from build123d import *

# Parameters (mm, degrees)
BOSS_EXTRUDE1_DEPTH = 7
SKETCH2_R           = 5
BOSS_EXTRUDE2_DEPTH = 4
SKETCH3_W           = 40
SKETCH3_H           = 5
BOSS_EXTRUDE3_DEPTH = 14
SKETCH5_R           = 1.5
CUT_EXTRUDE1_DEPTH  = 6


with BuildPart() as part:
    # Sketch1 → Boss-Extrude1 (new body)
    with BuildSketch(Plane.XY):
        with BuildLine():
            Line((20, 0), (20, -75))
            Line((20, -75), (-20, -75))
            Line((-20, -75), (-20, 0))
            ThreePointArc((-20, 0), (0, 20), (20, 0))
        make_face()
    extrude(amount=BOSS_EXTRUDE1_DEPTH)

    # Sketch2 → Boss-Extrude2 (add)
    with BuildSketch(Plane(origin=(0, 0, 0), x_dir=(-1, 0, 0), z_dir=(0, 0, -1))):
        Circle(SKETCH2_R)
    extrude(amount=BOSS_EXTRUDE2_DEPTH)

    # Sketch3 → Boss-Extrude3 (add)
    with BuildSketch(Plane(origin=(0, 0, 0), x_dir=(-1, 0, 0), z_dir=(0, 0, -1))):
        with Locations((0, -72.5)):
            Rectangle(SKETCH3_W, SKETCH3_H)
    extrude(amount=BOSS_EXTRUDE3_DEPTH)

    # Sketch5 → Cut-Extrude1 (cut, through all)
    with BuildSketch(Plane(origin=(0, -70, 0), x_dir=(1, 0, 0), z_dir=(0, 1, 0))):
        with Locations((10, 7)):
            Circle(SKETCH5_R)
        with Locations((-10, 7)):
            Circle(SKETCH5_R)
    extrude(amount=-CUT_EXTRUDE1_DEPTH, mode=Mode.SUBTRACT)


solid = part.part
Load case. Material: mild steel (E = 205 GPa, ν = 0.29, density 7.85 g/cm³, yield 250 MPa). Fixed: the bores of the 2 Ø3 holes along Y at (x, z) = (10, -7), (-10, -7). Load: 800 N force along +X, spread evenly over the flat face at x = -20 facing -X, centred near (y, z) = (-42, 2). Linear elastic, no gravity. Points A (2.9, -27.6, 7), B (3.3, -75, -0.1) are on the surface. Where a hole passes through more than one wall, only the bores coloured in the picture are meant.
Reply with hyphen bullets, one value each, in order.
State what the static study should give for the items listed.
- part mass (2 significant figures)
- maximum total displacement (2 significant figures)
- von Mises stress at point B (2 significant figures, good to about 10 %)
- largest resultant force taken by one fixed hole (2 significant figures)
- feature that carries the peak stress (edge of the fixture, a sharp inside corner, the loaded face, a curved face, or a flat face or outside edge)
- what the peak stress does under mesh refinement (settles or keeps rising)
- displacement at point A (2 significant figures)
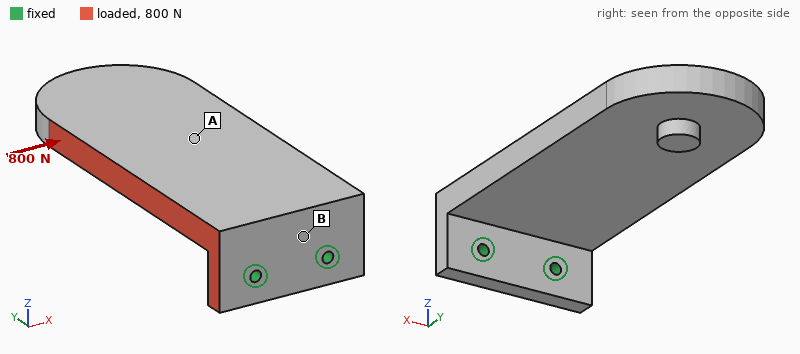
- 220 g
- 55 µm
- 28 MPa
- 1.2 kN
- edge of the fixture
- keeps rising
- 25 µm
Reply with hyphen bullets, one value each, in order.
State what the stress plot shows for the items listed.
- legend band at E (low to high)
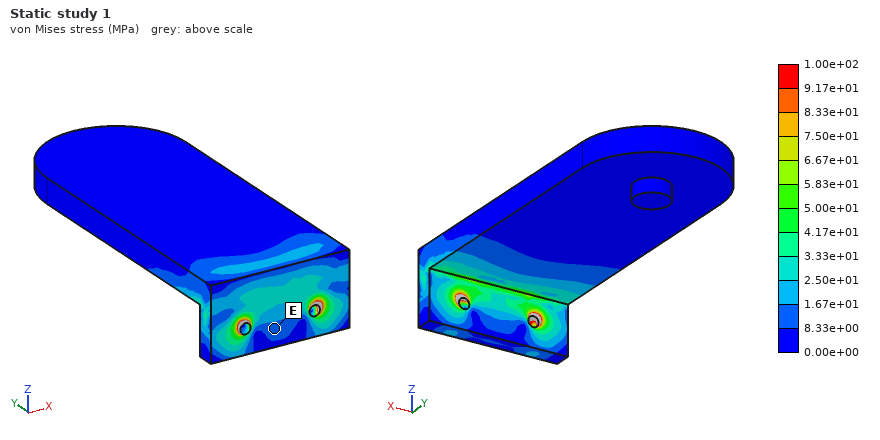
- 8.33e+00 to 1.67e+01 MPa
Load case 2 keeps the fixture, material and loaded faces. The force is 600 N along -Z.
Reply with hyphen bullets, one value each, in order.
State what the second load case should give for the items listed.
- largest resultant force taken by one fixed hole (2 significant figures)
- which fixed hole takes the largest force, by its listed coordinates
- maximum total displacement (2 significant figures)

- 850 N
- (-10, -7)
- 0.34 mm
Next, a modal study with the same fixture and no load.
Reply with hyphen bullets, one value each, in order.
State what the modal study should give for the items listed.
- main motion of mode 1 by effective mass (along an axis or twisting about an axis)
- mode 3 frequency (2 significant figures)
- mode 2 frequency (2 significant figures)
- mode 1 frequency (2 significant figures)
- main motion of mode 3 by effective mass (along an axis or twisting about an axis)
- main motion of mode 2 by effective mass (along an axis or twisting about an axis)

- along Z
- 3300 Hz
- 1400 Hz
- 480 Hz
- twisting about Y
- along X
